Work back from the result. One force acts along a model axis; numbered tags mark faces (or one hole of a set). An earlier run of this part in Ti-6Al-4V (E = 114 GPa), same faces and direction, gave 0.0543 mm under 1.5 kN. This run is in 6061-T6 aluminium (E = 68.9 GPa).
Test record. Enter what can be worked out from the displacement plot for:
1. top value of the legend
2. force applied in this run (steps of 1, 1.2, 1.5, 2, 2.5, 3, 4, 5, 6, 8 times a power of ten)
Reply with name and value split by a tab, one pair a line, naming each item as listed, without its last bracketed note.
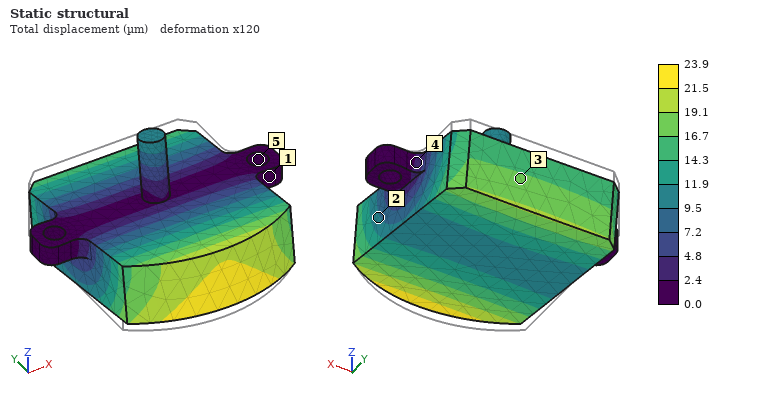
top value of the legend	23.9 µm
force applied in this run	400 N
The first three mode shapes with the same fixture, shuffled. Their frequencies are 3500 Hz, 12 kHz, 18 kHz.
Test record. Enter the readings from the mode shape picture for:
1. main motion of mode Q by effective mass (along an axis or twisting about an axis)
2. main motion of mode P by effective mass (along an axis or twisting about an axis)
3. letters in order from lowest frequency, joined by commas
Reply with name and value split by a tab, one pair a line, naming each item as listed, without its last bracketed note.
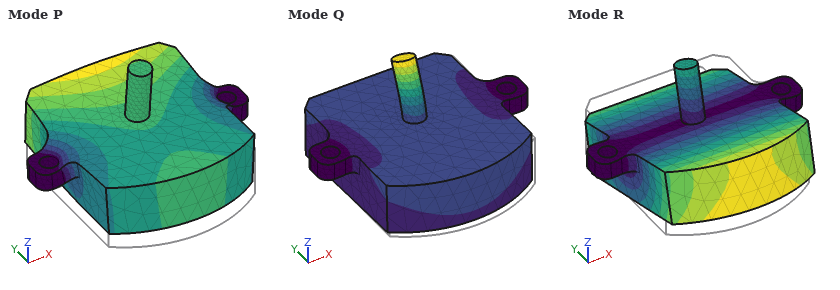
main motion of mode Q by effective mass	along Y
main motion of mode P by effective mass	along Z
letters in order from lowest frequency, joined by commas	R, P, Q
